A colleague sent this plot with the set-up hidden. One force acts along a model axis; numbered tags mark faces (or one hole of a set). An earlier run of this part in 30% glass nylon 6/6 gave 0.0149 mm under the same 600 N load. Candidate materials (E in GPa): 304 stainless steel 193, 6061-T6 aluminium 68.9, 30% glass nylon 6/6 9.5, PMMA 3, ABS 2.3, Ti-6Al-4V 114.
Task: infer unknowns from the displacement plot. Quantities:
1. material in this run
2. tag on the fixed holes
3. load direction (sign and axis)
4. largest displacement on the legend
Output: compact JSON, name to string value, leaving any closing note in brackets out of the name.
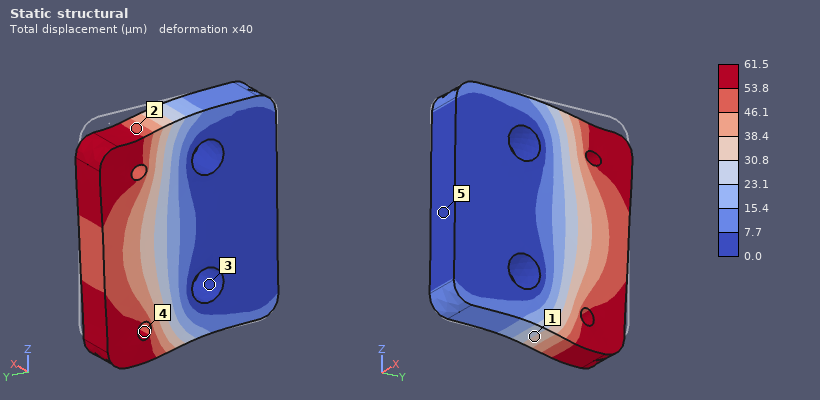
{"material in this run": "ABS", "tag on the fixed holes": "3", "load direction": "-Z", "largest displacement on the legend": "61.5 µm"}
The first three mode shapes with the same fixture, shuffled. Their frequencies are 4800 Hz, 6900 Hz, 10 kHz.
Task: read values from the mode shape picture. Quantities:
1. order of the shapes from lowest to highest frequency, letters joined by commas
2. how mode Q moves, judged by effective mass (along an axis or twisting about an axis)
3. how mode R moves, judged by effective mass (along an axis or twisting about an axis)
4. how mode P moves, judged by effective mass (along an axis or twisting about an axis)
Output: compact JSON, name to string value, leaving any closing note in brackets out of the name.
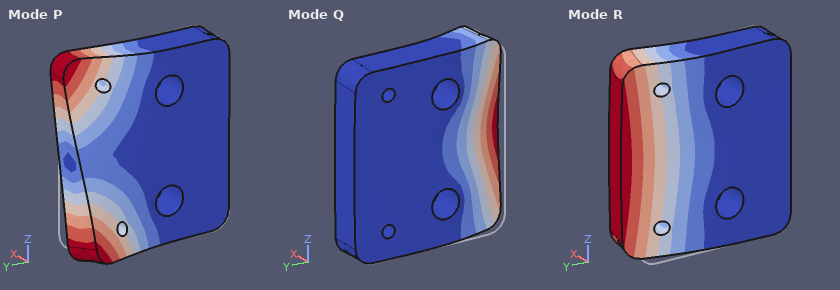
{"order of the shapes from lowest to highest frequency, letters joined by commas": "R, P, Q", "how mode Q moves, judged by effective mass": "along X", "how mode R moves, judged by effective mass": "along X", "how mode P moves, judged by effective mass": "twisting about Y"}
